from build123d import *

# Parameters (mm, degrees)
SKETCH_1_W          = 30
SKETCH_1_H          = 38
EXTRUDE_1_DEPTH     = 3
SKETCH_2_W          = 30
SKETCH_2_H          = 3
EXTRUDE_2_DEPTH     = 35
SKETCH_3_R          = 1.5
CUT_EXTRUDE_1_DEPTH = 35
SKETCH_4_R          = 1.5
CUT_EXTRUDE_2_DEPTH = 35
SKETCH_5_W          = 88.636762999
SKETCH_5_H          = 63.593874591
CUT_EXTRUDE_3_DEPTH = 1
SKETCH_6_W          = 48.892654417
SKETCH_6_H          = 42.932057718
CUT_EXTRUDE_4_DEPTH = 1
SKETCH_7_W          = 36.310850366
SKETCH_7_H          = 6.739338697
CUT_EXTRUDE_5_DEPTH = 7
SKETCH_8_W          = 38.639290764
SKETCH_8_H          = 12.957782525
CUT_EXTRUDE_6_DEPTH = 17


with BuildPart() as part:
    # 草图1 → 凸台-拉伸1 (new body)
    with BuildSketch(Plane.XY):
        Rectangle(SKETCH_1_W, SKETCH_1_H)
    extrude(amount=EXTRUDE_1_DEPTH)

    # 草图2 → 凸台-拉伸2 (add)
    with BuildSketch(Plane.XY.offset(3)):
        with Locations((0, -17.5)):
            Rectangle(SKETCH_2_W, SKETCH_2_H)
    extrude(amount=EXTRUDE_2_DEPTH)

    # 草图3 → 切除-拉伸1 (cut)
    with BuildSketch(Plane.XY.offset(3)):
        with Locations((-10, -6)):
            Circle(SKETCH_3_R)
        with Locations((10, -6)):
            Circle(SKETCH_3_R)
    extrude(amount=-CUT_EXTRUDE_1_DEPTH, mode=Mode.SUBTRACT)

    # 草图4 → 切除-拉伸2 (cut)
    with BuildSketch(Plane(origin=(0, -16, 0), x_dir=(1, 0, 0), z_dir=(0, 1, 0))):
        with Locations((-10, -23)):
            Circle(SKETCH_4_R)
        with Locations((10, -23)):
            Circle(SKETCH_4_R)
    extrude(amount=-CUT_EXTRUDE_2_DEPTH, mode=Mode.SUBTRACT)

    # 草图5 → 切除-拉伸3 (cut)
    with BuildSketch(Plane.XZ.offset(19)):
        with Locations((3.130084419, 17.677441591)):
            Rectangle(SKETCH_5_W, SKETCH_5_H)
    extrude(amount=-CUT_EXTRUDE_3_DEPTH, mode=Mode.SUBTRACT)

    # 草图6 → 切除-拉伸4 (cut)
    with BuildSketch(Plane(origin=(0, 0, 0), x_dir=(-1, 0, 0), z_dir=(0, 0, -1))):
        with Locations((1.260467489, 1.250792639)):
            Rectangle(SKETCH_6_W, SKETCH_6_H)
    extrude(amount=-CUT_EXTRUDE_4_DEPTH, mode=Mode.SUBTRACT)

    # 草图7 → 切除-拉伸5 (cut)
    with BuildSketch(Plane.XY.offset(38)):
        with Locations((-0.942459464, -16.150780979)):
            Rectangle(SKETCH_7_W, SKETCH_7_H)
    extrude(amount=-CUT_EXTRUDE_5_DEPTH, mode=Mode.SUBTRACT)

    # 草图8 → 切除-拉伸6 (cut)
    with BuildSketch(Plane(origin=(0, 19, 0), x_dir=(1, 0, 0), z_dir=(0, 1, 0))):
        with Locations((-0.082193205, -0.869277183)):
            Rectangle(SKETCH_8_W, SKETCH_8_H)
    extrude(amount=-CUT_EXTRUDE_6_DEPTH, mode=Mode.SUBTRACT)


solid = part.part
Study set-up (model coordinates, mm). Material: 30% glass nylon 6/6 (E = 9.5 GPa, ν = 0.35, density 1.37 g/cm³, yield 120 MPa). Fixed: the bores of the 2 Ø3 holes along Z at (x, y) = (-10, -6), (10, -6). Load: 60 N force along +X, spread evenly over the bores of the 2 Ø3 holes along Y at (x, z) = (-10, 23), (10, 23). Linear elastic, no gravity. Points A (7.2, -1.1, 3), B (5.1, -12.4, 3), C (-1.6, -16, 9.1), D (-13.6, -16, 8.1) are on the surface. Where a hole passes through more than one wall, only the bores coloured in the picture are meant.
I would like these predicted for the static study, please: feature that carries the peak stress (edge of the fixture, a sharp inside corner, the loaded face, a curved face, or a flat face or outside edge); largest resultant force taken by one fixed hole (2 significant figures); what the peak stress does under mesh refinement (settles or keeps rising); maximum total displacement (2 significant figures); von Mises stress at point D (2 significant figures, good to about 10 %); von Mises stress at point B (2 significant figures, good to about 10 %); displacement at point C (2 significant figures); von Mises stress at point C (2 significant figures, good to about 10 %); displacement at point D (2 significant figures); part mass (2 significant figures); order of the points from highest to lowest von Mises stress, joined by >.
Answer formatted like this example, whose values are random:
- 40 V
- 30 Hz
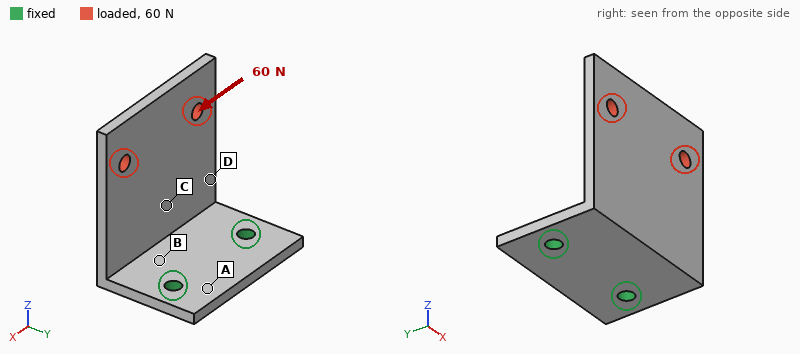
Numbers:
- edge of the fixture
- 72 N
- keeps rising
- 0.47 mm
- 15 MPa
- 21 MPa
- 0.10 mm
- 9.0 MPa
- 0.20 mm
- 3.9 g
- B > D > C > A
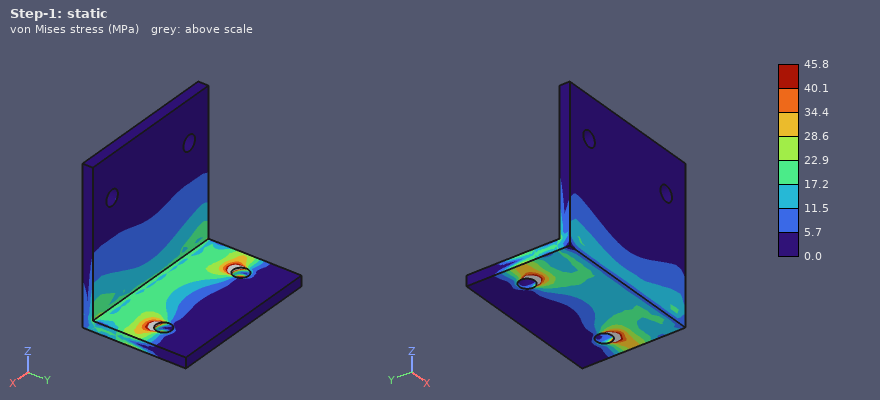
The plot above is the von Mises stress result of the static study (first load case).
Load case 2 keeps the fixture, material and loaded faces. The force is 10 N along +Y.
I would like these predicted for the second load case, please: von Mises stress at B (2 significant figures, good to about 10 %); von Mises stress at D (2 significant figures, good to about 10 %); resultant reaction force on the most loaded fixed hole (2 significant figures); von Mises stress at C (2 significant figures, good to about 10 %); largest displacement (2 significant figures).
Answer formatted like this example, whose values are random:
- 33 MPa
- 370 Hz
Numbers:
- 9.4 MPa
- 6.8 MPa
- 5.3 N
- 6.4 MPa
- 0.54 mm
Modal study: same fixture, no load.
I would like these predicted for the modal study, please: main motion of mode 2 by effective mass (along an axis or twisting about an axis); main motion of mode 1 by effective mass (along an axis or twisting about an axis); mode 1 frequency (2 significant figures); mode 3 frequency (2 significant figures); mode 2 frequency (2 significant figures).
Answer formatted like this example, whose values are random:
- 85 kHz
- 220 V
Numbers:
- along X
- along Y
- 670 Hz
- 2400 Hz
- 1600 Hz
